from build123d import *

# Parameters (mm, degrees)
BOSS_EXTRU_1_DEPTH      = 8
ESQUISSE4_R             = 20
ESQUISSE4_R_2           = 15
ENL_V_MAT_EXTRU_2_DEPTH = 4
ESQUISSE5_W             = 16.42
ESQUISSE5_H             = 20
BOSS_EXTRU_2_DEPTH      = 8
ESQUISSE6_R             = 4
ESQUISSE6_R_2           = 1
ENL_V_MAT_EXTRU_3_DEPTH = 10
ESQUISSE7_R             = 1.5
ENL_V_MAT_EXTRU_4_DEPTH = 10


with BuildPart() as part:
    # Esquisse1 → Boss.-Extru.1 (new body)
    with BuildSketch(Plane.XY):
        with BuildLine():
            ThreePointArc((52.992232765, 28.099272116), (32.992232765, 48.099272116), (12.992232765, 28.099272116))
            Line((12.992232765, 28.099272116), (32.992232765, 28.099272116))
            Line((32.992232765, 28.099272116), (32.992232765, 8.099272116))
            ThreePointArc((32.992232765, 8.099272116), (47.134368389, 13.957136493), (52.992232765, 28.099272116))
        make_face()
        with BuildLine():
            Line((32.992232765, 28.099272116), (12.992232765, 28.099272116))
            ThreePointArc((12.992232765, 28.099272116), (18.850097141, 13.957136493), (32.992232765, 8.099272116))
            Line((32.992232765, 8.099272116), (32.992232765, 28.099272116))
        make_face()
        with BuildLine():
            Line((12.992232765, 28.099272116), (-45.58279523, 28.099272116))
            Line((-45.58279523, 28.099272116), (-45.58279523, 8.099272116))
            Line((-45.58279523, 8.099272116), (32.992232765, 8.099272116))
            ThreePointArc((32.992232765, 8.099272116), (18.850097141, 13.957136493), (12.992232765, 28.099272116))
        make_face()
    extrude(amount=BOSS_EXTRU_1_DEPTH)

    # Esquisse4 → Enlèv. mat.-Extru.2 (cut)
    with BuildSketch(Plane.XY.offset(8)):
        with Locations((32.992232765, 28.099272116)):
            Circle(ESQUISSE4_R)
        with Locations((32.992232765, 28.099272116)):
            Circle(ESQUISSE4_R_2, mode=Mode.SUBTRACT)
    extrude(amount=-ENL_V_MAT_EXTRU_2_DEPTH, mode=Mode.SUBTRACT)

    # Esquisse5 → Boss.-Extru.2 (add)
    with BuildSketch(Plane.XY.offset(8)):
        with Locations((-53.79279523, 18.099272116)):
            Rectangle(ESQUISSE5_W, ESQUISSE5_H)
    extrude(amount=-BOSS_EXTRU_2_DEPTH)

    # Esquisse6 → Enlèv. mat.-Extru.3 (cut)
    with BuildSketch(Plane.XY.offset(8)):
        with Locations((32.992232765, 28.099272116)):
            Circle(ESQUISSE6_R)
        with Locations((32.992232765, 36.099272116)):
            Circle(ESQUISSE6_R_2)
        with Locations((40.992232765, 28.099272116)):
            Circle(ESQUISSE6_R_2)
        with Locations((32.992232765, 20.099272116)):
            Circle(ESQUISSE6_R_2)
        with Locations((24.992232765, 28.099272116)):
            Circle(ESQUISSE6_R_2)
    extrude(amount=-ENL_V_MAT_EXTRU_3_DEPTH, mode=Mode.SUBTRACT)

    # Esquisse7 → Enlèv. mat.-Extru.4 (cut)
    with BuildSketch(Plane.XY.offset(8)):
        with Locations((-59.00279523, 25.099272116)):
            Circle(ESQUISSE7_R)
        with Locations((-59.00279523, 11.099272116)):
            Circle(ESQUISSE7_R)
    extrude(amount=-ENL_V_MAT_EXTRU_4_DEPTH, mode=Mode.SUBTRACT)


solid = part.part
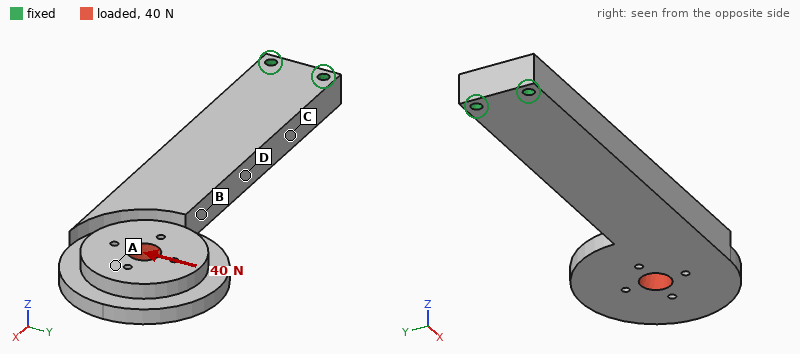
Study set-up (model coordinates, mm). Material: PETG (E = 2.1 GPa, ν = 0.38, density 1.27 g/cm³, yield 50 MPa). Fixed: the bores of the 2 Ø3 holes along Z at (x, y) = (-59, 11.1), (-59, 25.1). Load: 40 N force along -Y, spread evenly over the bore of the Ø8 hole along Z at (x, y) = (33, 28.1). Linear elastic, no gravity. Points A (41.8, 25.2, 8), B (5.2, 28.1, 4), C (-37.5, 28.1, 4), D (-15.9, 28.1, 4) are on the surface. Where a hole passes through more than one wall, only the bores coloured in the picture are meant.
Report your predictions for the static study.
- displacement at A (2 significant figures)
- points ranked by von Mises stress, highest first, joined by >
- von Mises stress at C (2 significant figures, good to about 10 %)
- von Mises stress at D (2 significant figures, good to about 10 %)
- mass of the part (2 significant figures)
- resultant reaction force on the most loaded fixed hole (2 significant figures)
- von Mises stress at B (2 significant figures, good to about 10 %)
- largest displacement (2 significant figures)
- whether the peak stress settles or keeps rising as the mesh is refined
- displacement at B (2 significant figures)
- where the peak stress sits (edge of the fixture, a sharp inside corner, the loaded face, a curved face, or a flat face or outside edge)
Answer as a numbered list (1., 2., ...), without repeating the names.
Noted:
1. 1.1 mm
2. C > D > B > A
3. 5.3 MPa
4. 3.7 MPa
5. 25 g
6. 250 N
7. 2.1 MPa
8. 1.3 mm
9. keeps rising
10. 0.55 mm
11. edge of the fixture
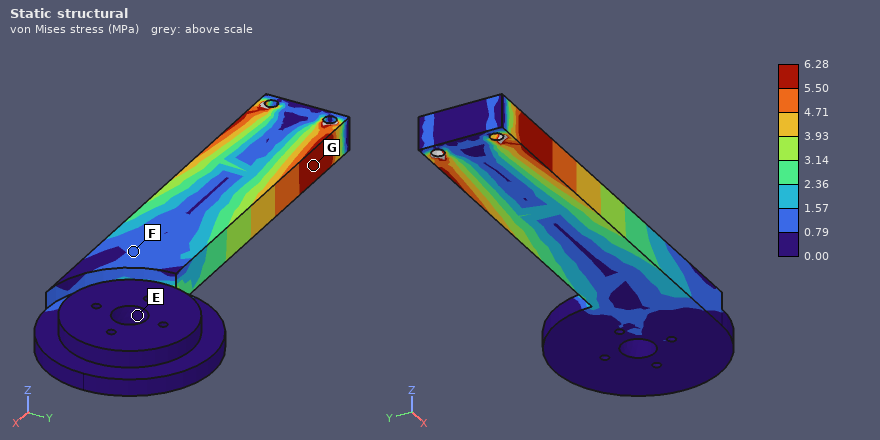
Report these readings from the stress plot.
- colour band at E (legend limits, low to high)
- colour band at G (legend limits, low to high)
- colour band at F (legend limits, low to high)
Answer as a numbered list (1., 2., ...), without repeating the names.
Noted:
1. 0.00 to 0.79 MPa
2. 5.50 to 6.28 MPa
3. 0.79 to 1.57 MPa
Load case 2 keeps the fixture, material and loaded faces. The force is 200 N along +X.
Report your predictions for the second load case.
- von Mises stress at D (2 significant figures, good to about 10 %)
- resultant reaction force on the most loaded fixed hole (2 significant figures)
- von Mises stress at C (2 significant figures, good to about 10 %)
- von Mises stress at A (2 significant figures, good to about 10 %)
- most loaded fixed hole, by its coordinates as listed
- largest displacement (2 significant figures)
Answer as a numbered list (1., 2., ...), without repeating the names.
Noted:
1. 5.0 MPa
2. 240 N
3. 5.0 MPa
4. 0.85 MPa
5. (-59, 25.1)
6. 1.2 mm
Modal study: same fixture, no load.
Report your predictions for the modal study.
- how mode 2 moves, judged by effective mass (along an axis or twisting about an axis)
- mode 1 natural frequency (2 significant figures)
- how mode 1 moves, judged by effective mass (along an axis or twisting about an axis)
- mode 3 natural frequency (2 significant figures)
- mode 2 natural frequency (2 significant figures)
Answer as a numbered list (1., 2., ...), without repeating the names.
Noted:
1. along Y
2. 120 Hz
3. along Z
4. 580 Hz
5. 300 Hz
